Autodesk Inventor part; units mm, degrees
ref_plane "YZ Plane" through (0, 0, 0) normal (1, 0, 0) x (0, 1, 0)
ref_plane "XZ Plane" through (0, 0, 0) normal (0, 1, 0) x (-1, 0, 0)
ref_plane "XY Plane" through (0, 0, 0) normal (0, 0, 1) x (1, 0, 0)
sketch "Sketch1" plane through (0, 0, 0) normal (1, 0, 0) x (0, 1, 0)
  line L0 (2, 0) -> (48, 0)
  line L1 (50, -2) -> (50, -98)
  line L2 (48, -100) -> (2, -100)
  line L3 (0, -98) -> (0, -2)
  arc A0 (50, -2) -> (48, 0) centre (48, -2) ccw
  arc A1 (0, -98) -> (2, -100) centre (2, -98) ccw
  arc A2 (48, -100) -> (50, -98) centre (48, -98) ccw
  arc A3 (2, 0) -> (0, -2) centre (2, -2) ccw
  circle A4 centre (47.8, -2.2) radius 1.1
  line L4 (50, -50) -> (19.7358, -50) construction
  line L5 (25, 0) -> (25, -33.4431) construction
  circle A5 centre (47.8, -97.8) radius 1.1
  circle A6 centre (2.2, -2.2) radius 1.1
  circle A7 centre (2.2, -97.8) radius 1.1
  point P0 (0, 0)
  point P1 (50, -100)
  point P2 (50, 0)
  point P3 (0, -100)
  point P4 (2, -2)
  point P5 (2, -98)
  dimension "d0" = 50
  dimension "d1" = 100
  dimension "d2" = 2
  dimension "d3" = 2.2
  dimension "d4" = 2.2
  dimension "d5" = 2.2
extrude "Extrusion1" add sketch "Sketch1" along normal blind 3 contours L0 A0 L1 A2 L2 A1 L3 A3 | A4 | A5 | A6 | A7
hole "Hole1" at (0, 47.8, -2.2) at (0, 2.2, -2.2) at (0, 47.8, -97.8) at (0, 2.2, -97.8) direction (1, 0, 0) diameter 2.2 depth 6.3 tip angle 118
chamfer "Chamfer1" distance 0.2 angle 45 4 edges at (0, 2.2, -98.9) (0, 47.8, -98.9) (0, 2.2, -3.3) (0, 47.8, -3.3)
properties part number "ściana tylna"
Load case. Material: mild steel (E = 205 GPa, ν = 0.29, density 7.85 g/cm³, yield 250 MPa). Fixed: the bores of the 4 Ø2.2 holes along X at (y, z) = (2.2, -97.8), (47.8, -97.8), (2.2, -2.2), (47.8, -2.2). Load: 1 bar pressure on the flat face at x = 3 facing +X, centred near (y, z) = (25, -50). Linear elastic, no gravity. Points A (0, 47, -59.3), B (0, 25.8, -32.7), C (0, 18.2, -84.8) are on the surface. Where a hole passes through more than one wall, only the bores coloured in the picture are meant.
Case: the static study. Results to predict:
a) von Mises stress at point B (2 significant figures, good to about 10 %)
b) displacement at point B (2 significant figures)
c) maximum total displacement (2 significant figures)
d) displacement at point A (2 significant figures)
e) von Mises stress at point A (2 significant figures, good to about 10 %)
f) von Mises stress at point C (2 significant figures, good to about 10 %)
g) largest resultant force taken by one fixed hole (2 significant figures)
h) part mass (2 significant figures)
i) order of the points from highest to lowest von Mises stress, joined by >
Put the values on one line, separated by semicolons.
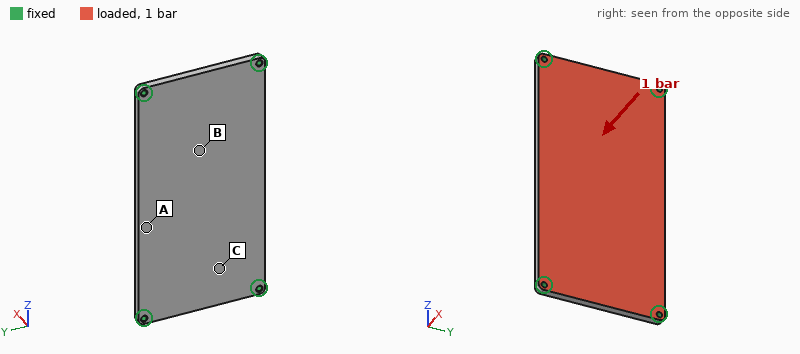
21 MPa; 64 µm; 80 µm; 74 µm; 33 MPa; 12 MPa; 120 N; 120 g; A > B > C
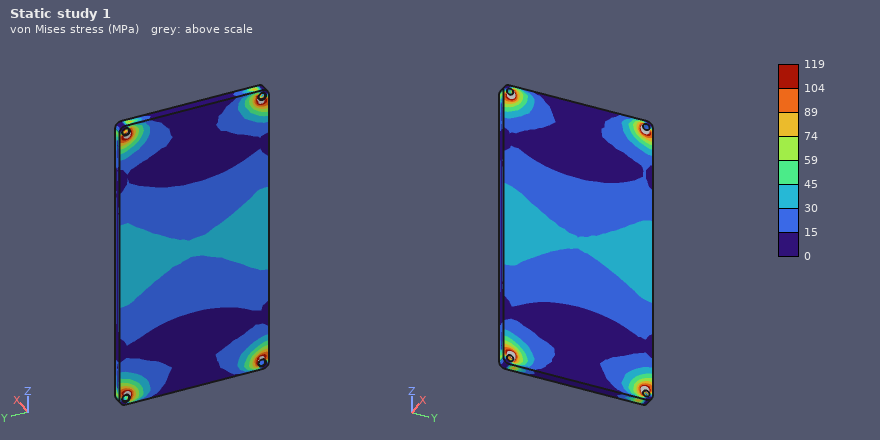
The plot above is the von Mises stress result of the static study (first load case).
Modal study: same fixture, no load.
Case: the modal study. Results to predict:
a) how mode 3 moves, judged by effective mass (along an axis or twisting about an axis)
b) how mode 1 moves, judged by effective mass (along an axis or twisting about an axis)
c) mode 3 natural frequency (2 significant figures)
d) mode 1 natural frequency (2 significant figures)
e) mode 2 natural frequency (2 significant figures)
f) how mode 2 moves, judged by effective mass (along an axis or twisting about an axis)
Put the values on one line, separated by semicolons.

twisting about Y; along X; 3800 Hz; 1300 Hz; 2700 Hz; twisting about Z
